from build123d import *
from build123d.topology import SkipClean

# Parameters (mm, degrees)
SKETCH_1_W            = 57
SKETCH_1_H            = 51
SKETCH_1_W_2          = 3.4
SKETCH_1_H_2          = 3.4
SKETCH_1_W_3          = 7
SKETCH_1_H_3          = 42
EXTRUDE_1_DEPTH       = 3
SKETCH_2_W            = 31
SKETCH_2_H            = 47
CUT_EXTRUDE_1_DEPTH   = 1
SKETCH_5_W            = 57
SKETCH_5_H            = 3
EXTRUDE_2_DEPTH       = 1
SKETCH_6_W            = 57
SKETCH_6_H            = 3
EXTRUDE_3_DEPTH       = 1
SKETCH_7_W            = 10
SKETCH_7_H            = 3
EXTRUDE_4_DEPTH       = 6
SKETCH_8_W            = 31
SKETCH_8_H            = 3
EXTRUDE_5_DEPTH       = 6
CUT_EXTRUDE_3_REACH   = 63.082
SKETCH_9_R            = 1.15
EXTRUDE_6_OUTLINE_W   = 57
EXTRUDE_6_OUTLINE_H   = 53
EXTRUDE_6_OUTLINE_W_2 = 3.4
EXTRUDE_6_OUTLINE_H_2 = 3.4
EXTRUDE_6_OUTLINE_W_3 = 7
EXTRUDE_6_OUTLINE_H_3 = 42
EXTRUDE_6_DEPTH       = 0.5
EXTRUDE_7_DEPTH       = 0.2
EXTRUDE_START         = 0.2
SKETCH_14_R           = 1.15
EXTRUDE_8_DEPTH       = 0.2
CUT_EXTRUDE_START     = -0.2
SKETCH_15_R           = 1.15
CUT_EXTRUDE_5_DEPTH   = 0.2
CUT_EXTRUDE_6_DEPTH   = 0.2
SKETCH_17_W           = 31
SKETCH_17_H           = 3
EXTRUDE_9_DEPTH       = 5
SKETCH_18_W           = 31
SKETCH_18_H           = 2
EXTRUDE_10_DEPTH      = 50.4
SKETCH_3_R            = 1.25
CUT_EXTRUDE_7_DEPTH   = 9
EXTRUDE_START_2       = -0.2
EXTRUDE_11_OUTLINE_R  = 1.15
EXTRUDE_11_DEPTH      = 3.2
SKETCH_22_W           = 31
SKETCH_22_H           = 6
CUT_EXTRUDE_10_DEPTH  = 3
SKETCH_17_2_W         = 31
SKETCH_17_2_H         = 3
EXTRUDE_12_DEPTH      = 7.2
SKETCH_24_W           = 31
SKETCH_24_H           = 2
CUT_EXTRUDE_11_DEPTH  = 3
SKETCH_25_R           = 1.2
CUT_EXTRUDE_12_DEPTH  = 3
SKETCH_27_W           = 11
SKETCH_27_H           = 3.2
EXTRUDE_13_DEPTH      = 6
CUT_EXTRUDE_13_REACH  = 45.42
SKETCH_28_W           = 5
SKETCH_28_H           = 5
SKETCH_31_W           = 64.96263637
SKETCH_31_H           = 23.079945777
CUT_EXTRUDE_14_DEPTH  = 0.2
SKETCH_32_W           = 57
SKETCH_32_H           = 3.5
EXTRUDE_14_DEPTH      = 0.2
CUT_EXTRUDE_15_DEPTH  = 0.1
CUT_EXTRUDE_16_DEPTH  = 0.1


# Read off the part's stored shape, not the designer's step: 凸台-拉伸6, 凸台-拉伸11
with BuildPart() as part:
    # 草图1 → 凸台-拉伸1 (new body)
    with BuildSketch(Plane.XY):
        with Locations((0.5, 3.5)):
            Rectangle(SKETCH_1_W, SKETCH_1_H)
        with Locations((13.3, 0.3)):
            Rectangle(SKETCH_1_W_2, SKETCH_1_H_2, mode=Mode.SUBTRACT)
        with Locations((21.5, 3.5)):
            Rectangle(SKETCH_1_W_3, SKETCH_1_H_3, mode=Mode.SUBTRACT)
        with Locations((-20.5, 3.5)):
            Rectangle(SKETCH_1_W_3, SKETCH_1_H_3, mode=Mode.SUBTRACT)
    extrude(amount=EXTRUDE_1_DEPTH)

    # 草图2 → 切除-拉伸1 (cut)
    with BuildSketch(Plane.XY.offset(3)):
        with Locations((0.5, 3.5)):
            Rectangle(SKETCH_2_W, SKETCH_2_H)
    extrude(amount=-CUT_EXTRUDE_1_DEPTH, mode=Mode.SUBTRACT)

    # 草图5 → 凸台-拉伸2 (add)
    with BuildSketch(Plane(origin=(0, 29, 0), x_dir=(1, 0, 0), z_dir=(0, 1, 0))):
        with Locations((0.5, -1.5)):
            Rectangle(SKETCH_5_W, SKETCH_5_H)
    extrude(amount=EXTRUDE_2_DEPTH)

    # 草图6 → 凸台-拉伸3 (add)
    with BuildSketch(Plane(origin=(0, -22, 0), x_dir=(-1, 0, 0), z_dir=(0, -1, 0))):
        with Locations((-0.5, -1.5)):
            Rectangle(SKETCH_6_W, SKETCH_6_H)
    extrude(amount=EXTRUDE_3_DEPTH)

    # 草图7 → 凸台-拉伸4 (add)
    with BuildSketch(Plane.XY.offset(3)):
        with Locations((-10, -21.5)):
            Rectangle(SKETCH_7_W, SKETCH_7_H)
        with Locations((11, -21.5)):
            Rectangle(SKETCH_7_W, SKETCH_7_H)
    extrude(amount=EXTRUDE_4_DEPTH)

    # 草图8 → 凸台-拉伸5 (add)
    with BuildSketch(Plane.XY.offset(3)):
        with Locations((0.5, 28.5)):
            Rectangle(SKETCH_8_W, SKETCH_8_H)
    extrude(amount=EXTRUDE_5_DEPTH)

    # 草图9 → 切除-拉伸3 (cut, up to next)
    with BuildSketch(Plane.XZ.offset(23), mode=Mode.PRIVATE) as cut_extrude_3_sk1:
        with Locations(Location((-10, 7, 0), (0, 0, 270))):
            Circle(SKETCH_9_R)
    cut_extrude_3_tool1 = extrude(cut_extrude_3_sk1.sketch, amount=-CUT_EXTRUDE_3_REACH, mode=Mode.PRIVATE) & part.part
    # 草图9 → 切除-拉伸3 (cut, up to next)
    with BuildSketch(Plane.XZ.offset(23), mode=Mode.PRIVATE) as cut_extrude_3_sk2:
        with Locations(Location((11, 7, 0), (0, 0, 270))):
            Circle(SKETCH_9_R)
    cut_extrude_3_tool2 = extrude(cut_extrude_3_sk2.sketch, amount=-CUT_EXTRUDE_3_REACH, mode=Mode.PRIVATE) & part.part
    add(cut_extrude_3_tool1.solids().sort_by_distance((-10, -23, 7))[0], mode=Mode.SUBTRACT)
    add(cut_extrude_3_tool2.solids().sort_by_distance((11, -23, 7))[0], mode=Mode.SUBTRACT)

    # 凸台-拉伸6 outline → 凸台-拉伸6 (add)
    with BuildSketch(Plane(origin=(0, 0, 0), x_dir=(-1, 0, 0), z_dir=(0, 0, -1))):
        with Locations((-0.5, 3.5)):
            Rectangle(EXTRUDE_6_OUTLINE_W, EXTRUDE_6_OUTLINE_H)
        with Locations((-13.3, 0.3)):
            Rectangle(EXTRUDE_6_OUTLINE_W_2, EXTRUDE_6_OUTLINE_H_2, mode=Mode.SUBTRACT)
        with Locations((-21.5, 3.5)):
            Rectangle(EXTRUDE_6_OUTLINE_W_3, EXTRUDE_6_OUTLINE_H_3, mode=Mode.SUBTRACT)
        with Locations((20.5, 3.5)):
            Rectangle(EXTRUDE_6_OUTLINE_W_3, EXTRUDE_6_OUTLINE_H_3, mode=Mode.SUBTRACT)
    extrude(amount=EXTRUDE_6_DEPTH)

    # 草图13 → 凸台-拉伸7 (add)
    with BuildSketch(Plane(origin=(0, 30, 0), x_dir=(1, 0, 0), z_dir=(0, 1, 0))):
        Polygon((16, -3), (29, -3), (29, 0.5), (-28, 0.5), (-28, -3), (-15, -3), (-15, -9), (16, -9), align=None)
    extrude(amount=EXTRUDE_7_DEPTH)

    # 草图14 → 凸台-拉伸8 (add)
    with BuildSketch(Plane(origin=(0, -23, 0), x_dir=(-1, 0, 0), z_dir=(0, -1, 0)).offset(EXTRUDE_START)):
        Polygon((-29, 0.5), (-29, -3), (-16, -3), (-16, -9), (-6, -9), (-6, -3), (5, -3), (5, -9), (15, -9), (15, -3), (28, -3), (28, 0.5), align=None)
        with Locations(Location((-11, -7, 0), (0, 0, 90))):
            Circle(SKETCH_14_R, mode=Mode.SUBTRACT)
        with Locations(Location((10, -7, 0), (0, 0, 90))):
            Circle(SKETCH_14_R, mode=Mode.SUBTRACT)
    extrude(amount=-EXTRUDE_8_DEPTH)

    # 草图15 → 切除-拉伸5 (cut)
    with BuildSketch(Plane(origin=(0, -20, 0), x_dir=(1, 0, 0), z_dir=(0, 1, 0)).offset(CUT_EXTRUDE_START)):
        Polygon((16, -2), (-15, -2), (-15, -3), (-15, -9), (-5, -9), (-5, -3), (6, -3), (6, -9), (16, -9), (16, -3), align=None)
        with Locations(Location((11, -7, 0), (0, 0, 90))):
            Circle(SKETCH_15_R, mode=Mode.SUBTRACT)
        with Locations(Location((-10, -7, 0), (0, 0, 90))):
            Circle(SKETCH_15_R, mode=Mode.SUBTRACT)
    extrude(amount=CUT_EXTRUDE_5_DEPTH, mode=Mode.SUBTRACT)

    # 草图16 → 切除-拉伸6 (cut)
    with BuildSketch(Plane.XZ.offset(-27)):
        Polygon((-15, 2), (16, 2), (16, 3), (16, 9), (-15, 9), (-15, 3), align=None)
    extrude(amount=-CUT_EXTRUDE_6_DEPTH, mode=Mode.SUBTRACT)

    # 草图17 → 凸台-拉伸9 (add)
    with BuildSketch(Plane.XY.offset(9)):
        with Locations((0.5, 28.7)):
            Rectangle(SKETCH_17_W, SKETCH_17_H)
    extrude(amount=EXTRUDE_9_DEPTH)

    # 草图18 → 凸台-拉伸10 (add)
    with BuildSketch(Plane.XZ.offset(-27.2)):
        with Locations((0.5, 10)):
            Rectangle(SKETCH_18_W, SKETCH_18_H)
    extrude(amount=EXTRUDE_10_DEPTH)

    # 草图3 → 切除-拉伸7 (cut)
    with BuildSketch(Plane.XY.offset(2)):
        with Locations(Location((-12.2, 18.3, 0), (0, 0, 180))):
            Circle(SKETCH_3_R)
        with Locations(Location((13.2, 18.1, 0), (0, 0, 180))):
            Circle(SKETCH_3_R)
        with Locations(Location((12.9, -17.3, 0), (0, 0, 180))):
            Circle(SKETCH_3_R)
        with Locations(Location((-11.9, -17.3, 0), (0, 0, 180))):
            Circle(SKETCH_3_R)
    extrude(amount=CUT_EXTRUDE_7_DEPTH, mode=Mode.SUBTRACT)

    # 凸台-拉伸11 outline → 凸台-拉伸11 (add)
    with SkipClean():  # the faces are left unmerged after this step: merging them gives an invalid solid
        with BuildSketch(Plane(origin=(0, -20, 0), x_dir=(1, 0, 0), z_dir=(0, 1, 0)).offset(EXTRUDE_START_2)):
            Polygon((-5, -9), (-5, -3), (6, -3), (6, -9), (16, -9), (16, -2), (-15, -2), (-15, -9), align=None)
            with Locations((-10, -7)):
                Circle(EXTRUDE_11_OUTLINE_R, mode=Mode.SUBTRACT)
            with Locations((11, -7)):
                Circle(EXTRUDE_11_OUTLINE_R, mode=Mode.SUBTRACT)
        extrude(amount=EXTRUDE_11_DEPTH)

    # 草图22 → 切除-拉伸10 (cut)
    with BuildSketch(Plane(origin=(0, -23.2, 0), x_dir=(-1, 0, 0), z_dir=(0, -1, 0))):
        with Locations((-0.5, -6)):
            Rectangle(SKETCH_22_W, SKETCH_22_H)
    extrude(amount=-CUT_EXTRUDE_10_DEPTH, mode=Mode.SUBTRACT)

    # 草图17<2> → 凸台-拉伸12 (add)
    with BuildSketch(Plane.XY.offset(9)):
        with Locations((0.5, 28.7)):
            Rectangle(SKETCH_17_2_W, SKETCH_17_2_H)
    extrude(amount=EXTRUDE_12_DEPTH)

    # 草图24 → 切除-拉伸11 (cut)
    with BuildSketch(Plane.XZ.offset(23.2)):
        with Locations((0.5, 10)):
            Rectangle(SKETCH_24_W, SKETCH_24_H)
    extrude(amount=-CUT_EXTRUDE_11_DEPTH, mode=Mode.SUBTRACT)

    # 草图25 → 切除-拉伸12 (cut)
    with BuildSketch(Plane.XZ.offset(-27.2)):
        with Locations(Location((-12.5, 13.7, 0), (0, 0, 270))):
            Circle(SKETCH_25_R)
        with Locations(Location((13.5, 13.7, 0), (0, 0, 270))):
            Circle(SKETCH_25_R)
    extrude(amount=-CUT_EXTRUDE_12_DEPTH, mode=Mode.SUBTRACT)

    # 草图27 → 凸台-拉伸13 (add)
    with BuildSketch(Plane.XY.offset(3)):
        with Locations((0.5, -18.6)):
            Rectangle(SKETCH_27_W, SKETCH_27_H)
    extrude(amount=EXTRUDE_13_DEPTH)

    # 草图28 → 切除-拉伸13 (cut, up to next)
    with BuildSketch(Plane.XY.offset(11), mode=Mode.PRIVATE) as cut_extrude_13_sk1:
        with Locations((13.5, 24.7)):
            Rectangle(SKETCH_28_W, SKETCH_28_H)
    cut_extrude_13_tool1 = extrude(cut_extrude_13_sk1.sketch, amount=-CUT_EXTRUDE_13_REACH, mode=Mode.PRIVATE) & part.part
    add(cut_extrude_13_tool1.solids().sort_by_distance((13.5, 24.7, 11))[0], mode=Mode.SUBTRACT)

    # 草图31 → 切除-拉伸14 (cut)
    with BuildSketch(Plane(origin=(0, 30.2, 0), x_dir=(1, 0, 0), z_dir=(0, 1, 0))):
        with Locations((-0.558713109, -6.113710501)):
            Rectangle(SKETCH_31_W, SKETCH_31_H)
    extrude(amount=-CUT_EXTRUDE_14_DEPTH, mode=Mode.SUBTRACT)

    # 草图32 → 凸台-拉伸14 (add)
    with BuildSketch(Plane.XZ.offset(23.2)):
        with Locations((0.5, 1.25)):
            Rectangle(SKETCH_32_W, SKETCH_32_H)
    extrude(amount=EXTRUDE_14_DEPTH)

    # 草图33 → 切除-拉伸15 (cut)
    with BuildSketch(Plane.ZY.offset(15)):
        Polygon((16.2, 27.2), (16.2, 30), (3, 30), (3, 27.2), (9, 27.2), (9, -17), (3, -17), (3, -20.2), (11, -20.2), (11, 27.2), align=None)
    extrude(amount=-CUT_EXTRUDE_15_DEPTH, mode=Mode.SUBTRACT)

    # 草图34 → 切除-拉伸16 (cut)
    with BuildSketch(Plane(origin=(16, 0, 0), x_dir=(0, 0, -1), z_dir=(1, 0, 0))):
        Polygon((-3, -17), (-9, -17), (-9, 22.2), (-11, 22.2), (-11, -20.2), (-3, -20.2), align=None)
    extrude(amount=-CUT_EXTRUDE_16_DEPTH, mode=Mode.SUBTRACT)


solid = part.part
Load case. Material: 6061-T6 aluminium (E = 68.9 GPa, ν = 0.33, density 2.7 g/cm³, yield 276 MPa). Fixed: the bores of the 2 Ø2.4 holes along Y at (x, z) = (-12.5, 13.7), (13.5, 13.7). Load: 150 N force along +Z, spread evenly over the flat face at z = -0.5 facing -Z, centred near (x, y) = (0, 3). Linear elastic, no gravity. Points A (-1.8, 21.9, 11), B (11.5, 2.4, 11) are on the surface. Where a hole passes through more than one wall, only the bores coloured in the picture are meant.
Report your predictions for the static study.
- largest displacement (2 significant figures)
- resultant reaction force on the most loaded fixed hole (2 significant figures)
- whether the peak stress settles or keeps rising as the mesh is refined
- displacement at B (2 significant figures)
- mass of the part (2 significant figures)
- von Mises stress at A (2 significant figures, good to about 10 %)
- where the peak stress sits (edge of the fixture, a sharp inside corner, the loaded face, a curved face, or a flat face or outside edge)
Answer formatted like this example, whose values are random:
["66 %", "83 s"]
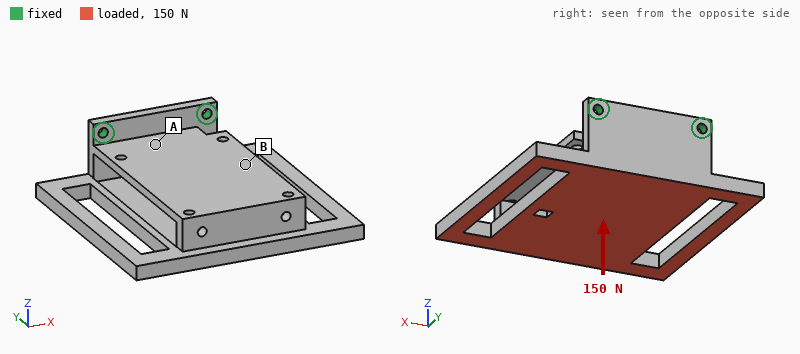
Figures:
["0.62 mm", "79 N", "keeps rising", "0.30 mm", "32 g", "33 MPa", "edge of the fixture"]
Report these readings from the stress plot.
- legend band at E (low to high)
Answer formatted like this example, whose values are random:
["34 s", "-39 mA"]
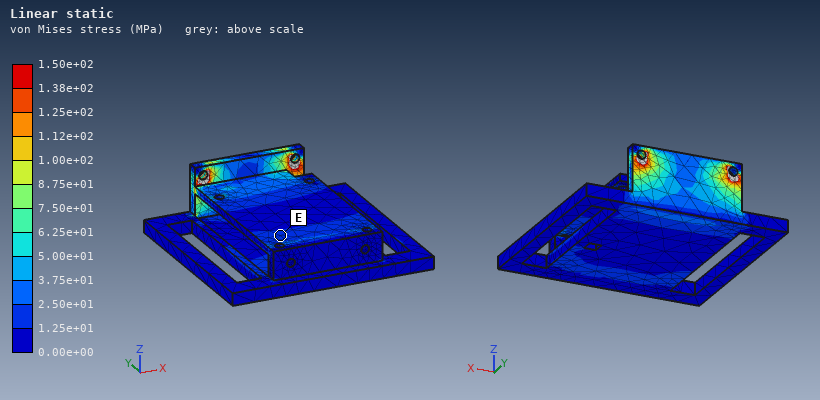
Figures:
["1.25e+01 to 2.50e+01 MPa"]
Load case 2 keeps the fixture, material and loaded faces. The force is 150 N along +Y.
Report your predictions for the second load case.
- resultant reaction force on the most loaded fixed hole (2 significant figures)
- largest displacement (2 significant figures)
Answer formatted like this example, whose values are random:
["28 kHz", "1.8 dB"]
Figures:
["79 N", "0.23 mm"]
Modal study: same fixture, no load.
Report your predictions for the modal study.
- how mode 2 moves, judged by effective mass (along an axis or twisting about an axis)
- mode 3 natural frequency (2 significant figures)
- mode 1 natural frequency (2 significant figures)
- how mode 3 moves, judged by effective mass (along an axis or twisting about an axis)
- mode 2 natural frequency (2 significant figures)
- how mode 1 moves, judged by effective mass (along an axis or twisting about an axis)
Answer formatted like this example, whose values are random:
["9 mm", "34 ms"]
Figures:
["along X", "2500 Hz", "530 Hz", "along X", "1900 Hz", "along Z"]
